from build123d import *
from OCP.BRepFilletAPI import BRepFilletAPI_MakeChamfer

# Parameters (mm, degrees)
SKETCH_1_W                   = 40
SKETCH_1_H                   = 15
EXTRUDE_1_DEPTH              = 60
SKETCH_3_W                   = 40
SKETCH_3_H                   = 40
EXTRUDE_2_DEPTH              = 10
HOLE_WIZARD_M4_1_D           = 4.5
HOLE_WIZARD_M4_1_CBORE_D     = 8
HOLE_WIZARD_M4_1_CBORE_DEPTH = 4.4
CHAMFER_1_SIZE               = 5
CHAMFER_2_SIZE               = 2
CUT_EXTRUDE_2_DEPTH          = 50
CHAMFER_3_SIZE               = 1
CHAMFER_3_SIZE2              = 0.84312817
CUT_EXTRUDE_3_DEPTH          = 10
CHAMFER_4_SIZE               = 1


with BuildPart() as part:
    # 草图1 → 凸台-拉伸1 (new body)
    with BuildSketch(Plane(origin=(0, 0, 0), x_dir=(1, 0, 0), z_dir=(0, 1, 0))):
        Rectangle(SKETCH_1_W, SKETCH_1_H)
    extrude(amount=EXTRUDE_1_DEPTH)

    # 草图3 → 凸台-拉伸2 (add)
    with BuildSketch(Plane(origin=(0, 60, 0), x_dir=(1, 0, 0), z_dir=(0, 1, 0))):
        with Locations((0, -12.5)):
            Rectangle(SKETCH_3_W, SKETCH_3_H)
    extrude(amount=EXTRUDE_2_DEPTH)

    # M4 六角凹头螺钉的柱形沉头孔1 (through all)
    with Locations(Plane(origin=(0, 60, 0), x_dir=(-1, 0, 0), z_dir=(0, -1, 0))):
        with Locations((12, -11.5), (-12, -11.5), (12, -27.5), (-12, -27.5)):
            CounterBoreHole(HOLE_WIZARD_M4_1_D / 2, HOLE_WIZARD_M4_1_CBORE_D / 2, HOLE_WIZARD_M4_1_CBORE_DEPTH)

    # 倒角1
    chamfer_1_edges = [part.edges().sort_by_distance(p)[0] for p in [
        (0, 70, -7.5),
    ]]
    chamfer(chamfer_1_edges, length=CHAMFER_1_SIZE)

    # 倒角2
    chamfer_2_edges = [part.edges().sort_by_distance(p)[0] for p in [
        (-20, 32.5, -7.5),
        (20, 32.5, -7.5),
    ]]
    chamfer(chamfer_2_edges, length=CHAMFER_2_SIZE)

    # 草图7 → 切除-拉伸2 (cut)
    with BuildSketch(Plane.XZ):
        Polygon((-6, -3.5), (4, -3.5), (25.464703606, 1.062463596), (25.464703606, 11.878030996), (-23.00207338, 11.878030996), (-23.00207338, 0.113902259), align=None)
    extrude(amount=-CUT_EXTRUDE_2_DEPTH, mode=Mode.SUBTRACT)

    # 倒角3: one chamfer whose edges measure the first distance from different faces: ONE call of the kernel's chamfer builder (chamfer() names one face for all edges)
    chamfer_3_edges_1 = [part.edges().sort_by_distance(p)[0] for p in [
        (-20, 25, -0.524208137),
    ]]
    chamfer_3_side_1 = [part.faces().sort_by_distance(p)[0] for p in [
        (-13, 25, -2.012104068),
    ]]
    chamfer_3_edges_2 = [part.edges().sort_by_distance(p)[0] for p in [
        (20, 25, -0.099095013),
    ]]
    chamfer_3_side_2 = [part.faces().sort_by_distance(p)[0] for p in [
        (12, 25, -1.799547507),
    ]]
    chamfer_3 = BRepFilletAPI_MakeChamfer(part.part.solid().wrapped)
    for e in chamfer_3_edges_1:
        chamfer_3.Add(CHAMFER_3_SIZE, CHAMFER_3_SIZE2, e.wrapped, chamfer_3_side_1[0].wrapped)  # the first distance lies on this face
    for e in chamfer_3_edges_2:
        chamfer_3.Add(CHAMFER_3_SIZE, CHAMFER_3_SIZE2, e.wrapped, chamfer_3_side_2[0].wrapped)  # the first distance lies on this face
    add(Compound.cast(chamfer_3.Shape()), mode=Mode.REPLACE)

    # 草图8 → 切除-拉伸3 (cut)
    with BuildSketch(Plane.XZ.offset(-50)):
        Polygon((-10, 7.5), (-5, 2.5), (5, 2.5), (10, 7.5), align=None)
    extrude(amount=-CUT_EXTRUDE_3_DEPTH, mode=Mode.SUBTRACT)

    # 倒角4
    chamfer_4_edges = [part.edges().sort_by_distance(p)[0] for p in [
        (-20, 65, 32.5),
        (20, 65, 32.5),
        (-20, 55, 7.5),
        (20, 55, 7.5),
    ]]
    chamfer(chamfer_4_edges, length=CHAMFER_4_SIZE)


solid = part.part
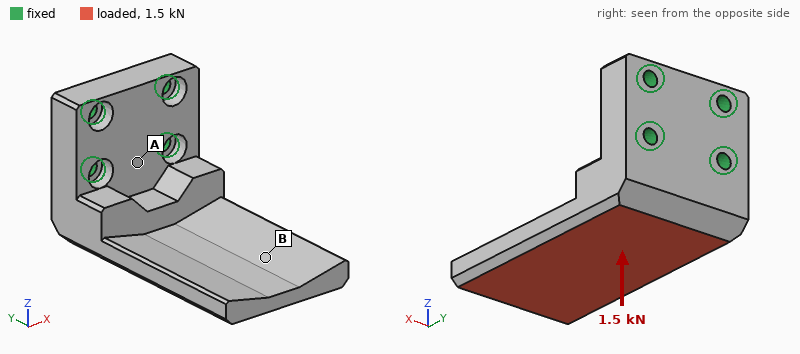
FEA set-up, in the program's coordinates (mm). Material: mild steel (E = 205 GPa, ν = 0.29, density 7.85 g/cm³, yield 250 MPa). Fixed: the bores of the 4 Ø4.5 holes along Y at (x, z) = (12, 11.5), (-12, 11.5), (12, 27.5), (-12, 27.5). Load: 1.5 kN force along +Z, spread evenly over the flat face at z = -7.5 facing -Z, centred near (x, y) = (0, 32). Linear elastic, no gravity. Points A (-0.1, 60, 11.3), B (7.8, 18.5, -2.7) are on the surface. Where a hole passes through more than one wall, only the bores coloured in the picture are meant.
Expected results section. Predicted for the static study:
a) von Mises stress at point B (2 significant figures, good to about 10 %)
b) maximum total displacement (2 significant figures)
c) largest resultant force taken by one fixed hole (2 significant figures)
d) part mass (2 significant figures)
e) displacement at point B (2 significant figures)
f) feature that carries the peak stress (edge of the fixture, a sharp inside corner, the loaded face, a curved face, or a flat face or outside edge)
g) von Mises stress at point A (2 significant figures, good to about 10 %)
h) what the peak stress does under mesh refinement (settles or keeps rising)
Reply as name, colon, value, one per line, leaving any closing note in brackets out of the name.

von Mises stress at point B: 18 MPa
maximum total displacement: 0.29 mm
largest resultant force taken by one fixed hole: 1.5 kN
part mass: 230 g
displacement at point B: 0.17 mm
feature that carries the peak stress: edge of the fixture
von Mises stress at point A: 63 MPa
what the peak stress does under mesh refinement: keeps rising
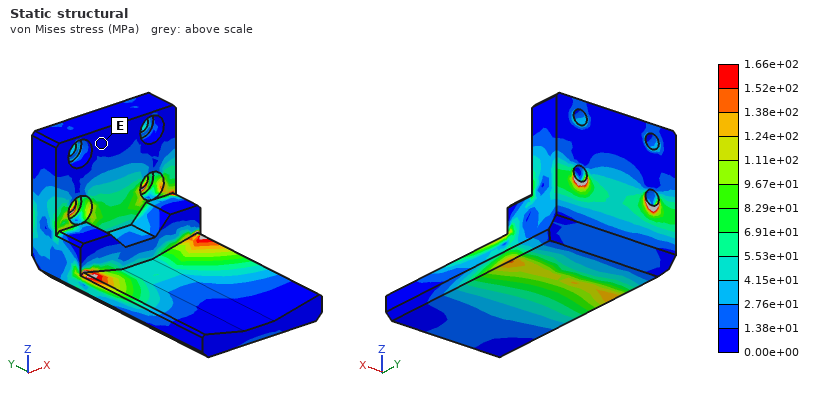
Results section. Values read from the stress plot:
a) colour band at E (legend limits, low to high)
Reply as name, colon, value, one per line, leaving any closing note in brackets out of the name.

colour band at E: 0.00e+00 to 1.38e+01 MPa
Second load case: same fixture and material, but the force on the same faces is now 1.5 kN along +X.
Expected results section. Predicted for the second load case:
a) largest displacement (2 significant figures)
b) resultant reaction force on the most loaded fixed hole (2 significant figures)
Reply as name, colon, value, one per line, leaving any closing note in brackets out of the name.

largest displacement: 29 µm
resultant reaction force on the most loaded fixed hole: 2.2 kN
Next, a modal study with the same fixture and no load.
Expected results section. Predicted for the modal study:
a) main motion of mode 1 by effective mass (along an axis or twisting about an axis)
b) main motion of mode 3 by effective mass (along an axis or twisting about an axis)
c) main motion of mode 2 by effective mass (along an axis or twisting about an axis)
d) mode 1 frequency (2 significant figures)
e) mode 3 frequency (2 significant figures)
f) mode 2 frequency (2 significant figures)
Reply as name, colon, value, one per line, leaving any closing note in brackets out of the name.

main motion of mode 1 by effective mass: along Z
main motion of mode 3 by effective mass: along X
main motion of mode 2 by effective mass: along X
mode 1 frequency: 1400 Hz
mode 3 frequency: 4700 Hz
mode 2 frequency: 3600 Hz
